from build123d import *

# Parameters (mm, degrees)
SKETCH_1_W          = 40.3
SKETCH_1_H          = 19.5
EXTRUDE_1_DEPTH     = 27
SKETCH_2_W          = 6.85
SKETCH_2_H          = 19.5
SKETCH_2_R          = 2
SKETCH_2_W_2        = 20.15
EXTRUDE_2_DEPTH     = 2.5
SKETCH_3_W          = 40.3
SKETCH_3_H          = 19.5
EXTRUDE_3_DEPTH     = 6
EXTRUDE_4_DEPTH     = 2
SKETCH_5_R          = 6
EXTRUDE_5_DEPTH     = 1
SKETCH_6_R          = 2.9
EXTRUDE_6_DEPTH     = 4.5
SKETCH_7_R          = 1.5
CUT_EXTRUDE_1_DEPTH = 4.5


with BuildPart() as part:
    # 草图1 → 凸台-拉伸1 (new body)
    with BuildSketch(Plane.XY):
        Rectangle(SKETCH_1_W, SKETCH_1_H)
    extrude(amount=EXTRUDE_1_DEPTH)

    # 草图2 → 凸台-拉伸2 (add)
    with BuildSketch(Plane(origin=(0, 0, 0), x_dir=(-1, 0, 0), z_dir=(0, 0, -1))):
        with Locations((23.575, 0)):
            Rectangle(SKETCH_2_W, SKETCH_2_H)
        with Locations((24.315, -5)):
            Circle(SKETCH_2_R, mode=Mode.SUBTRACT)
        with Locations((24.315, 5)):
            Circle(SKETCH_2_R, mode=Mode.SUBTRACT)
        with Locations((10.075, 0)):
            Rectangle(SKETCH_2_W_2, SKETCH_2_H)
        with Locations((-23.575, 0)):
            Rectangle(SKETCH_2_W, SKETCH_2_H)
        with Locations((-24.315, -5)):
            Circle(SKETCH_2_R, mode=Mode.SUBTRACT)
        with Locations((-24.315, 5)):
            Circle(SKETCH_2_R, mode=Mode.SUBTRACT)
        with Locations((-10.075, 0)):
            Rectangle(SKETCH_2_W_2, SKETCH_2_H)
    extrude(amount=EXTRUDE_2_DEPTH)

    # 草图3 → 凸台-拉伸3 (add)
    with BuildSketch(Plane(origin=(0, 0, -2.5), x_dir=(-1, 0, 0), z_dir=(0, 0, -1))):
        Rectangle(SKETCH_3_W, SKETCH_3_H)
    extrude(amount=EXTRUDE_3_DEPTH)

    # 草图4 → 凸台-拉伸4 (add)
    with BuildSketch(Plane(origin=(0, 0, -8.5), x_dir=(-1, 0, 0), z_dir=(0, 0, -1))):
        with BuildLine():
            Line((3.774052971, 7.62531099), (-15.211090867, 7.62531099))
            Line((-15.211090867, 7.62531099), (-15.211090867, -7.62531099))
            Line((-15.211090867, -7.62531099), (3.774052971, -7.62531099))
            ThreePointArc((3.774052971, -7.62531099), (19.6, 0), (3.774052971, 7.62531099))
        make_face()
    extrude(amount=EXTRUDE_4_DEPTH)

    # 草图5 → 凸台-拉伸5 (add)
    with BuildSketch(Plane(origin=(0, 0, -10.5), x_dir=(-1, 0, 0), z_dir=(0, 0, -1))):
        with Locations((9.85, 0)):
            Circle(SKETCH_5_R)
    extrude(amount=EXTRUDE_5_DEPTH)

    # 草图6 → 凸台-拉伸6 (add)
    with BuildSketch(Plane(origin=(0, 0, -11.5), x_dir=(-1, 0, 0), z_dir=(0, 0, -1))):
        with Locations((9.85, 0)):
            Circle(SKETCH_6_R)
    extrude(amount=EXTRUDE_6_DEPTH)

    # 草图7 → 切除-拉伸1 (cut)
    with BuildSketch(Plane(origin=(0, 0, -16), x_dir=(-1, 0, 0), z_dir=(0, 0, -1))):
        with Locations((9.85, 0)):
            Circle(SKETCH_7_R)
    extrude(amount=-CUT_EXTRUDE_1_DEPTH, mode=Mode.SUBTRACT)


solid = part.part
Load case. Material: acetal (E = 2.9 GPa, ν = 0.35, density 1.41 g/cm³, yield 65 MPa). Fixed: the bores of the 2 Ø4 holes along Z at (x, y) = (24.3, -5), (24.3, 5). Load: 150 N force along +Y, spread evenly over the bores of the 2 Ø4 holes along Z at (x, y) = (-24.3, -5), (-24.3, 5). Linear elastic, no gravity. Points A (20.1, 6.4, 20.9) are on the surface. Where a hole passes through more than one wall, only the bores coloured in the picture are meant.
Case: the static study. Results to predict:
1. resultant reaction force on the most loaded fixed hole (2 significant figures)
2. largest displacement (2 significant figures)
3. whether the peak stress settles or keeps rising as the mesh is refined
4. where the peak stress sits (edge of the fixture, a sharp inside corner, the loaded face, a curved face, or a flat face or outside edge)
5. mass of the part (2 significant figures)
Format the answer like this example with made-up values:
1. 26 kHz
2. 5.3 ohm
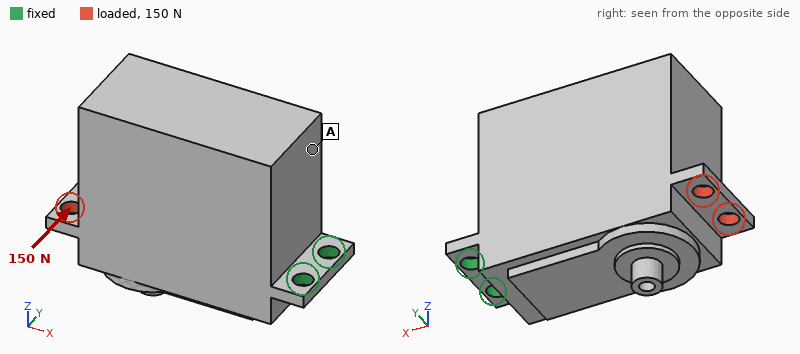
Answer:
1. 590 N
2. 0.69 mm
3. keeps rising
4. edge of the fixture
5. 42 g
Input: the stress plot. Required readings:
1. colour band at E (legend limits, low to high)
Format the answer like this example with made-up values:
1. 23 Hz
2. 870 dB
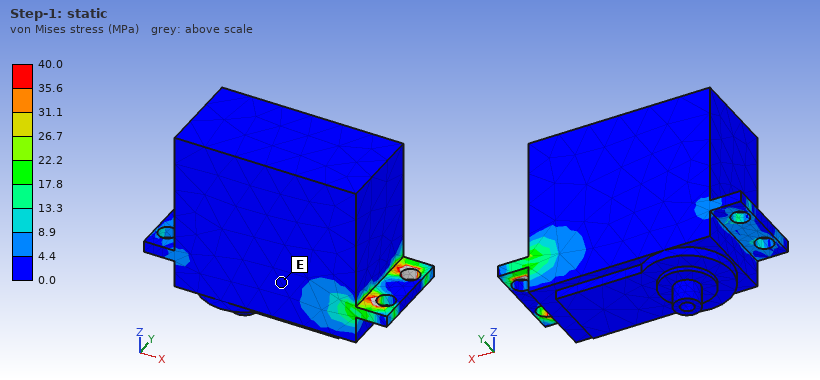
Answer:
1. 0.0 to 4.4 MPa
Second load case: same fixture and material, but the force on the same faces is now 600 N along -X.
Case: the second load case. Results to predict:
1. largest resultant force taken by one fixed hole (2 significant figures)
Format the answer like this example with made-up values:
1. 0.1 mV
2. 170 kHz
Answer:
1. 300 N
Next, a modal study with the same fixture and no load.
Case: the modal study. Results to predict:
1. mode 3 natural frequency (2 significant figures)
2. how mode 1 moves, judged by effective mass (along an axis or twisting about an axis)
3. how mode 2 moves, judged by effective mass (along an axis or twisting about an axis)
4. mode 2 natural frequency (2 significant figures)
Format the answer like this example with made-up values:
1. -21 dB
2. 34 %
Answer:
1. 1000 Hz
2. along Z
3. along Y
4. 580 Hz
